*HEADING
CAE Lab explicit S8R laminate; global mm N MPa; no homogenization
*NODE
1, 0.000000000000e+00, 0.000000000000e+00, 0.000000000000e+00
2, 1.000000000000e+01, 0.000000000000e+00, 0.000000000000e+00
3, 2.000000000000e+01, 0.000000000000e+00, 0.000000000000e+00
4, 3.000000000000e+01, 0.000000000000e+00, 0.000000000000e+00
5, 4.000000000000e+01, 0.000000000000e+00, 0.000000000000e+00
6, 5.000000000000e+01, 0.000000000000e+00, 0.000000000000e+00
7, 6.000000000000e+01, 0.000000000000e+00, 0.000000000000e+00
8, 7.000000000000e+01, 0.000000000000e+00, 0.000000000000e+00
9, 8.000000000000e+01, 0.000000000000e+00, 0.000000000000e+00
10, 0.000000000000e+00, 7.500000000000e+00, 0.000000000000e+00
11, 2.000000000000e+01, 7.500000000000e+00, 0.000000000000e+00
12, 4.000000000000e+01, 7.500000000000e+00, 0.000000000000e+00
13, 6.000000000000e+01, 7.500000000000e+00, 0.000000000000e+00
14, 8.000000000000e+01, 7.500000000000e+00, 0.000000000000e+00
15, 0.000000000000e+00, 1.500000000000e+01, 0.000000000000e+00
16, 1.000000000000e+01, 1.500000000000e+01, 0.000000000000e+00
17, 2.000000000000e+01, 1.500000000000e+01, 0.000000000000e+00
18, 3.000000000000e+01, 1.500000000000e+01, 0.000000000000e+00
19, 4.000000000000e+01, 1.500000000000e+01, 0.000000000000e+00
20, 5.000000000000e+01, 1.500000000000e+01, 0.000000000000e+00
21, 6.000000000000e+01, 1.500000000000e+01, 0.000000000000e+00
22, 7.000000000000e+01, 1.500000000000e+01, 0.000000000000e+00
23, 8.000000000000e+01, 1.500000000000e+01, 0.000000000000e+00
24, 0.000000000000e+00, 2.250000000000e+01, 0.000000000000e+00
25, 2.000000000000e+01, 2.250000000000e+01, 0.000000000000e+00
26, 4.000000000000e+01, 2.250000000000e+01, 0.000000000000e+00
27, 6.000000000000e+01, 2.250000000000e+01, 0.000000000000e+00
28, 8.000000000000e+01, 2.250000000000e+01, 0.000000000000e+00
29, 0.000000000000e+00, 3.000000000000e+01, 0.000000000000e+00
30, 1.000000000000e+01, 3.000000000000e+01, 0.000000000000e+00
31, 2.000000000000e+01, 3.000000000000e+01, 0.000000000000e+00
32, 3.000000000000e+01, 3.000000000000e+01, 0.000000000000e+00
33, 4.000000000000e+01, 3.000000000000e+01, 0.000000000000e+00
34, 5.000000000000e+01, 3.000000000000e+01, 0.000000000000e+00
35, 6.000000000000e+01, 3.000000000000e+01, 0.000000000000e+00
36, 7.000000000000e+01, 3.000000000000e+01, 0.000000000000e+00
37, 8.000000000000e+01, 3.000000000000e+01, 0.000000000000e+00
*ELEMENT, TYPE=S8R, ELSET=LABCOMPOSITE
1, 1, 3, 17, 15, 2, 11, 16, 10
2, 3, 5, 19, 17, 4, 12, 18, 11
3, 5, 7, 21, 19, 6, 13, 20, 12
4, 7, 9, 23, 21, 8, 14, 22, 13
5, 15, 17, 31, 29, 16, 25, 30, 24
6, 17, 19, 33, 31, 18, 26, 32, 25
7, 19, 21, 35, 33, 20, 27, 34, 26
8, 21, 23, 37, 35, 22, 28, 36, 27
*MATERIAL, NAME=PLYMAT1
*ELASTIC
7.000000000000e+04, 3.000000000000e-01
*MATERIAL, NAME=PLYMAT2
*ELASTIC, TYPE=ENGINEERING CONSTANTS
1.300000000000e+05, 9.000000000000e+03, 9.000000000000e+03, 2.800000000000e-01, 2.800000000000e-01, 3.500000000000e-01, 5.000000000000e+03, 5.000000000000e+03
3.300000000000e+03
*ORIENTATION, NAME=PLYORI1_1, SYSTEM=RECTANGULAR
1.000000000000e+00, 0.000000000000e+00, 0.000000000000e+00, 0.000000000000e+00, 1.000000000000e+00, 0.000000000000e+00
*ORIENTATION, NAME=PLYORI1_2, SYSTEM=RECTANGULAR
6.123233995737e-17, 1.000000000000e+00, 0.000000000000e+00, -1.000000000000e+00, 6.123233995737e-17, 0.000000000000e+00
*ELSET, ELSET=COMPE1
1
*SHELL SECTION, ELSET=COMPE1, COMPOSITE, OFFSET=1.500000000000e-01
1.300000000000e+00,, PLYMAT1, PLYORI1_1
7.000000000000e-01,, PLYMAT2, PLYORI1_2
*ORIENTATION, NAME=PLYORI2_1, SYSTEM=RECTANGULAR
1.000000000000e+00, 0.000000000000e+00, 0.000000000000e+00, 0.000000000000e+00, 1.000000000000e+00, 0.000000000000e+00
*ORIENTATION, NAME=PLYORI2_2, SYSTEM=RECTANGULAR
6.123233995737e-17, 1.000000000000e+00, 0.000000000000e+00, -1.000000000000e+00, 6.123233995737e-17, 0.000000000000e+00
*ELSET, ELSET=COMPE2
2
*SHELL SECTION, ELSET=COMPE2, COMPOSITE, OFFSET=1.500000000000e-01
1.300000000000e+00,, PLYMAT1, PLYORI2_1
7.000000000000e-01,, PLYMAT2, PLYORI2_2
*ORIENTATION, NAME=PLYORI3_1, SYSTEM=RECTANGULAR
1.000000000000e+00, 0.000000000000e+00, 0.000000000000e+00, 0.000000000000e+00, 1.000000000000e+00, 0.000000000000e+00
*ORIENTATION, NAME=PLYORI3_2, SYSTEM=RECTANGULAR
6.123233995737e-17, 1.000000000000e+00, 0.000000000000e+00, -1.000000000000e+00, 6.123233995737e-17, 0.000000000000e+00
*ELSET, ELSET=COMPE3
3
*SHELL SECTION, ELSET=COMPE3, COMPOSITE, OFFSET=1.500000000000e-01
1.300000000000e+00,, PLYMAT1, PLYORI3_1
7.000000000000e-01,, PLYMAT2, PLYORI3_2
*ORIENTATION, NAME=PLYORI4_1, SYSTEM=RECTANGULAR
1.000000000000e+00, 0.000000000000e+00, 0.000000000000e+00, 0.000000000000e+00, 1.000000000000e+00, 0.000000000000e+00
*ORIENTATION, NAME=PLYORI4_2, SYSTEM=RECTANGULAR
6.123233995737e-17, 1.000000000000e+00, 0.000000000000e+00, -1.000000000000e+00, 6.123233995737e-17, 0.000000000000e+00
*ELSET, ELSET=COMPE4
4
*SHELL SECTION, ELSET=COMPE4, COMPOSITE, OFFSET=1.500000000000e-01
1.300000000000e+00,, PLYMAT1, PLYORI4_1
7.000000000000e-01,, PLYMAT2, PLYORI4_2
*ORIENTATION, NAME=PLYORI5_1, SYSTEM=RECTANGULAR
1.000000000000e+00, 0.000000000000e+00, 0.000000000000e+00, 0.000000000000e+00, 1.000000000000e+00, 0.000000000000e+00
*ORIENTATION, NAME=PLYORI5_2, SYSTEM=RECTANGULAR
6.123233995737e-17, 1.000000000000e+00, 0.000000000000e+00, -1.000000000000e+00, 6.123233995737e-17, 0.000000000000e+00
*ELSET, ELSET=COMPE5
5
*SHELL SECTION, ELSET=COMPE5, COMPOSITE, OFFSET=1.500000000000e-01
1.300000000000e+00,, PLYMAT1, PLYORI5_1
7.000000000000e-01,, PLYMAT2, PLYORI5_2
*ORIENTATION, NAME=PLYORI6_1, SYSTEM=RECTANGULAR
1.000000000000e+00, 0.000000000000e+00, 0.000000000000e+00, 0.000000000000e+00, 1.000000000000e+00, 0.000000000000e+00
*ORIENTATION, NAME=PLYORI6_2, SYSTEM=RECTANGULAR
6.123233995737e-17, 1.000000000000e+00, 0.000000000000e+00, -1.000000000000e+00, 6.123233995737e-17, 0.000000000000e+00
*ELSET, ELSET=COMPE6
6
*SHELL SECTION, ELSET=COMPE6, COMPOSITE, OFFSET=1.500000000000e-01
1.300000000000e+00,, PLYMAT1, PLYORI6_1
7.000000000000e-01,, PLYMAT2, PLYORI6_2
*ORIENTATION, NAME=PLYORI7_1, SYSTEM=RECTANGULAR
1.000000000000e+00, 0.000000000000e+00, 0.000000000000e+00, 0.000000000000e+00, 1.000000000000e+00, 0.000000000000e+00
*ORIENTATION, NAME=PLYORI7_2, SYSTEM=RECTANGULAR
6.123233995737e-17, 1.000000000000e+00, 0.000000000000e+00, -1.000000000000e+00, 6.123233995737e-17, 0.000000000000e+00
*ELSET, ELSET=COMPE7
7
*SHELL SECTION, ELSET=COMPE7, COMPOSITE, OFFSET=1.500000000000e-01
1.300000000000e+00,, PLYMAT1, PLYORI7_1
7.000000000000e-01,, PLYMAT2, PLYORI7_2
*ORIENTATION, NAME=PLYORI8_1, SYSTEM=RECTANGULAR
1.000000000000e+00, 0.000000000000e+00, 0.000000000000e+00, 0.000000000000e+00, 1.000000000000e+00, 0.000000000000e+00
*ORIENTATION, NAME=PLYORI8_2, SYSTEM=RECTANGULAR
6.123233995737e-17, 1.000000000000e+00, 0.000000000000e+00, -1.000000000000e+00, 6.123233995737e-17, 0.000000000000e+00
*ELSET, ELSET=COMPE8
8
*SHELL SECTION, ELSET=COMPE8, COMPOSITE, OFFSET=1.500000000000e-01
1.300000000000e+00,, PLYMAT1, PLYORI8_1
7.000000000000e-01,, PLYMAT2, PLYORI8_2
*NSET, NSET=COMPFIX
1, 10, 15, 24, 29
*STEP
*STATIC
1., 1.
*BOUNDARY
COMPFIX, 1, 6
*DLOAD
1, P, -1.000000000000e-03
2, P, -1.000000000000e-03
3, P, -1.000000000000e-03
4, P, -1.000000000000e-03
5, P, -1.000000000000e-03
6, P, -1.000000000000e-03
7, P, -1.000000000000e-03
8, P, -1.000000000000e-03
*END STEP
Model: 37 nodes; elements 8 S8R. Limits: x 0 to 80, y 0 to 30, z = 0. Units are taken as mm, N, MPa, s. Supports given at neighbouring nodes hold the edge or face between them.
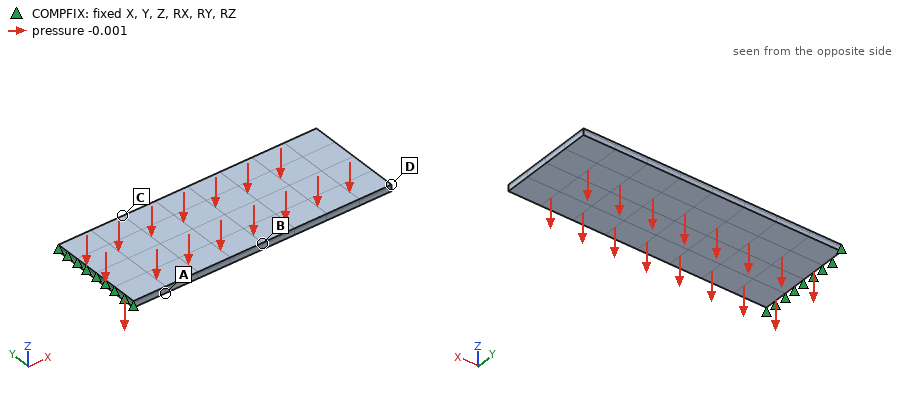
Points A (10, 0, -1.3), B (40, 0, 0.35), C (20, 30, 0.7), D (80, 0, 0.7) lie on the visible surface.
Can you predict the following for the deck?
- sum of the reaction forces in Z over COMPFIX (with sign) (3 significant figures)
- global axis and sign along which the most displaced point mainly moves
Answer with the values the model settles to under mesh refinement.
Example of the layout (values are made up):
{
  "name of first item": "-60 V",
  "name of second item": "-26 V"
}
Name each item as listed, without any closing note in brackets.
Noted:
{
  "sum of the reaction forces in Z over COMPFIX (with sign)": "2.40 N",
  "global axis and sign along which the most displaced point mainly moves": "-Z"
}
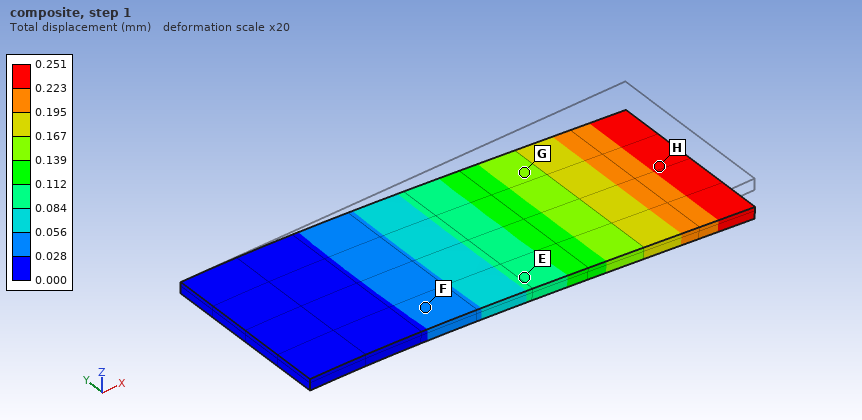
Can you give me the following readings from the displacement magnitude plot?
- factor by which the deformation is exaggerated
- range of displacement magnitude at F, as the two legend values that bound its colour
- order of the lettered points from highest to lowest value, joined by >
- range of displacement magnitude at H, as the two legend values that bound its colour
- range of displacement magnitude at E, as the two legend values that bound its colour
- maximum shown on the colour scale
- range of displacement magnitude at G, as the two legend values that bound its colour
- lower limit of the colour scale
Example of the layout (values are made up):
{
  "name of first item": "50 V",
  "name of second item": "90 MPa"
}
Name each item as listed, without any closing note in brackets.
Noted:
{
  "factor by which the deformation is exaggerated": "20",
  "range of displacement magnitude at F, as the two legend values that bound its colour": "0.028 to 0.056 mm",
  "order of the lettered points from highest to lowest value, joined by >": "H > G > E > F",
  "range of displacement magnitude at H, as the two legend values that bound its colour": "0.223 to 0.251 mm",
  "range of displacement magnitude at E, as the two legend values that bound its colour": "0.084 to 0.112 mm",
  "maximum shown on the colour scale": "0.251 mm",
  "range of displacement magnitude at G, as the two legend values that bound its colour": "0.139 to 0.167 mm",
  "lower limit of the colour scale": "0.000 mm"
}
